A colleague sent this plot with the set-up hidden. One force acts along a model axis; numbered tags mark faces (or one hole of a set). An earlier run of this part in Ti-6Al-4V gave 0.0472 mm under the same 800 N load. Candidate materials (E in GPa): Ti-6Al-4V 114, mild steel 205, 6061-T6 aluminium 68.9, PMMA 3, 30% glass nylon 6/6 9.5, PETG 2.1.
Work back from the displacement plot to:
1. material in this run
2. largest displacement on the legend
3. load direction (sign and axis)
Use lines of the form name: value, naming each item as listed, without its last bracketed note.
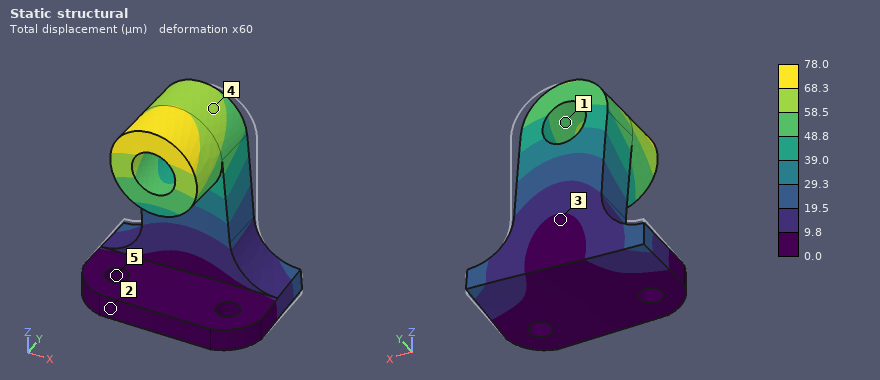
material in this run: 6061-T6 aluminium
largest displacement on the legend: 78.0 µm
load direction: -X
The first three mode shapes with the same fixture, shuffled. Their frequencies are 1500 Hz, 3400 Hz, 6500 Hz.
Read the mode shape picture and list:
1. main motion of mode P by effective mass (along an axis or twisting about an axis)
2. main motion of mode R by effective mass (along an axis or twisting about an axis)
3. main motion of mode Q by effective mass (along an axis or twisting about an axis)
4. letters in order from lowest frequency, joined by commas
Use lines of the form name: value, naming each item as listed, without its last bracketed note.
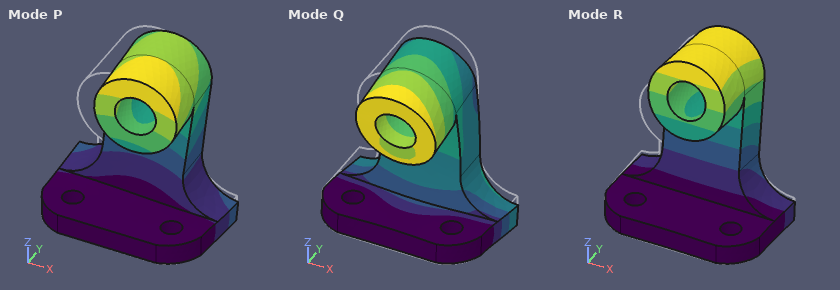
main motion of mode P by effective mass: along X
main motion of mode R by effective mass: along Y
main motion of mode Q by effective mass: along Z
letters in order from lowest frequency, joined by commas: R, P, Q
